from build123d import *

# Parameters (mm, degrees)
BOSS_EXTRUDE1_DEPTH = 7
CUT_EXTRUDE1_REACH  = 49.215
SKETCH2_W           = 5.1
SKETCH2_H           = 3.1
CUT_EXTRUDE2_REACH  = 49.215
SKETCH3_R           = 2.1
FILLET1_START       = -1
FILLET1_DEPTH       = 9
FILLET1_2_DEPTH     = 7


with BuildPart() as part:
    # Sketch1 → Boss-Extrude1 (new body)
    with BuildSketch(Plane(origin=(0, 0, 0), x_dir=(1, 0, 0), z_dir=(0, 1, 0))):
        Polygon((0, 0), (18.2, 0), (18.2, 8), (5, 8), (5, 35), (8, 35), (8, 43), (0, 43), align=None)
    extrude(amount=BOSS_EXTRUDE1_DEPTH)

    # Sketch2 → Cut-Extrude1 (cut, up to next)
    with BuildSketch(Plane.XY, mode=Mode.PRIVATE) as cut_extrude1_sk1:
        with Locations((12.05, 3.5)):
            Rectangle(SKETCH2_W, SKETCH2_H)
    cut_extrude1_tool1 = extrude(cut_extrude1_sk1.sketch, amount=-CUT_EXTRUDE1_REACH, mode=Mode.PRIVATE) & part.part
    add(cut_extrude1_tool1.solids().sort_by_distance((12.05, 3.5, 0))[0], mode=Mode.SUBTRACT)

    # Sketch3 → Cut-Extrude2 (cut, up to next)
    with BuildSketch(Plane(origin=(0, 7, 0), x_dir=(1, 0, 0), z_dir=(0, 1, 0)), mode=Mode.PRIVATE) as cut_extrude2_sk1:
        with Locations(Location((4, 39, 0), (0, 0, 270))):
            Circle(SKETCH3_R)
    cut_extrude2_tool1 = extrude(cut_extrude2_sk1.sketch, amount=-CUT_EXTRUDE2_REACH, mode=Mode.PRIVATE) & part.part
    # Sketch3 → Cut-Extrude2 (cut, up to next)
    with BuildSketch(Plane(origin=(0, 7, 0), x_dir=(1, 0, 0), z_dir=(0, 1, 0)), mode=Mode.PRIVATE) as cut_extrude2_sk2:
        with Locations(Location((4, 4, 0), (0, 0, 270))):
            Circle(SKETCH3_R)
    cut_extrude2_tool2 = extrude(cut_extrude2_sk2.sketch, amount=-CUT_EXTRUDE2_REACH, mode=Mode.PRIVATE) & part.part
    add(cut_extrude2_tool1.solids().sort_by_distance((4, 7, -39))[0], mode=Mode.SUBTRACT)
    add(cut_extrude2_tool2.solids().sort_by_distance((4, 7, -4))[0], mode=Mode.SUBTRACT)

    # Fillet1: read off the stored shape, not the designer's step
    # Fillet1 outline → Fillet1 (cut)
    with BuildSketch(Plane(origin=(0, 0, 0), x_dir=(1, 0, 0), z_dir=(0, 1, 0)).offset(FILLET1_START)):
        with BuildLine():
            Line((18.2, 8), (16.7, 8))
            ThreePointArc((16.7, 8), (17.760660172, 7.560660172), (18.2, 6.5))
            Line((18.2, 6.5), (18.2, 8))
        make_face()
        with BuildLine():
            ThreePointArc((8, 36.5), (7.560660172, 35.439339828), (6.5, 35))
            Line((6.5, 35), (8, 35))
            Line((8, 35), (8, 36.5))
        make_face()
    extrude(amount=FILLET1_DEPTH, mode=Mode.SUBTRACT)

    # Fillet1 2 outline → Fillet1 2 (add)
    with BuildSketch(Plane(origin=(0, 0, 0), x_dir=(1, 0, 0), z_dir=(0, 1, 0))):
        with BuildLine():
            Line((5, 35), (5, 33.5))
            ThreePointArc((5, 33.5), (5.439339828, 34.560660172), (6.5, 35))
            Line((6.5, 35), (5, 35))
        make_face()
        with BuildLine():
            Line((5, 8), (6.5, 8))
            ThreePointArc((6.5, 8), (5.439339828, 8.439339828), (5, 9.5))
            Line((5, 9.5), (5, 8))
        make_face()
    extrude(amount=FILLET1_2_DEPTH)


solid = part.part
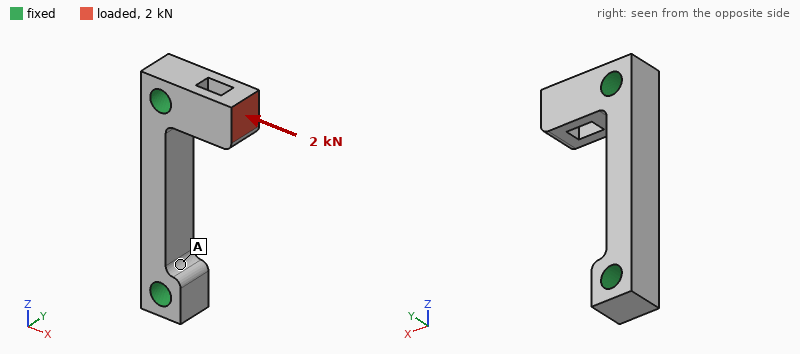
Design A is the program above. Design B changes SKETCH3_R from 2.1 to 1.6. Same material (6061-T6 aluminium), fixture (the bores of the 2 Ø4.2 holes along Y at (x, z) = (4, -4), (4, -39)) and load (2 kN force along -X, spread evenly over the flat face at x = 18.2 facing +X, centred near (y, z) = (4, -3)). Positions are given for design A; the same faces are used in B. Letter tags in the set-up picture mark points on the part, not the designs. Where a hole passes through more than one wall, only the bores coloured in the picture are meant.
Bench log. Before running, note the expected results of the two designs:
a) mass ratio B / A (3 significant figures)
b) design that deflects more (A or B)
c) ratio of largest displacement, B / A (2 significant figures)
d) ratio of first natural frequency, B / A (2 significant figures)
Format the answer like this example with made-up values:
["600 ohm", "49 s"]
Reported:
["1.04", "B", "1.1", "0.96"]
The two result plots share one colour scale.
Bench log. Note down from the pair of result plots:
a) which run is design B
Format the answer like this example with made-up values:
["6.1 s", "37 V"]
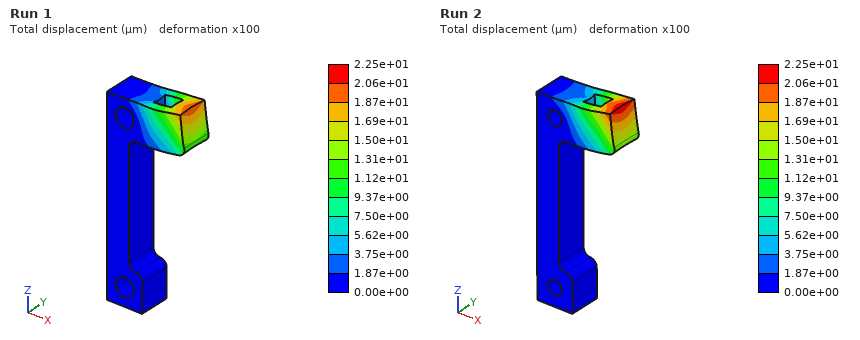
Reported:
["Run 2"]
